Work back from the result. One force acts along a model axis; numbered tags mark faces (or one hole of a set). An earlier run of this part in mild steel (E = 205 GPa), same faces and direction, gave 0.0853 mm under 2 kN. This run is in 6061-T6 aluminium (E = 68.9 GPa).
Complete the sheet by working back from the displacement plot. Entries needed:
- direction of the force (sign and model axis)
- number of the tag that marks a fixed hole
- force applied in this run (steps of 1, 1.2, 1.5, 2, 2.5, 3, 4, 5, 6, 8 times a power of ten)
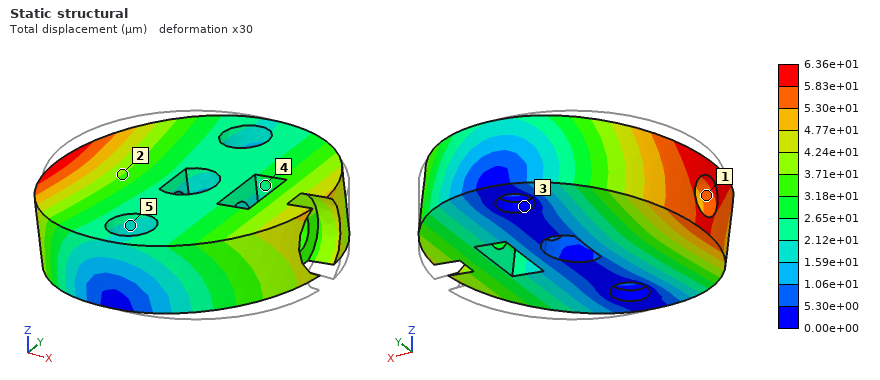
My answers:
-Z
3
500 N
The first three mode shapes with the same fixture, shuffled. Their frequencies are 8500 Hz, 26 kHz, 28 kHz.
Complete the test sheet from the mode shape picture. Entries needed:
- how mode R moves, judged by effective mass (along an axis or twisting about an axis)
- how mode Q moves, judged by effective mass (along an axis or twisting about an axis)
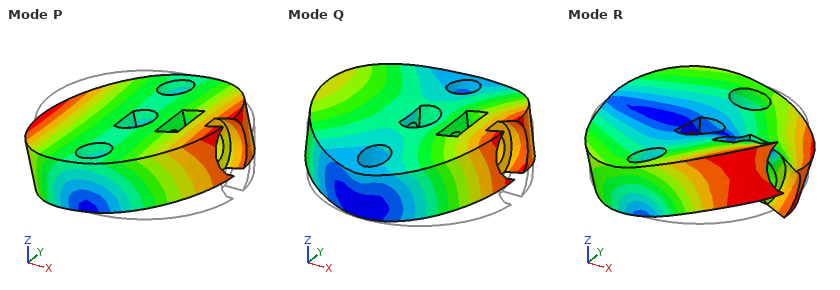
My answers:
twisting about Z
along Z
